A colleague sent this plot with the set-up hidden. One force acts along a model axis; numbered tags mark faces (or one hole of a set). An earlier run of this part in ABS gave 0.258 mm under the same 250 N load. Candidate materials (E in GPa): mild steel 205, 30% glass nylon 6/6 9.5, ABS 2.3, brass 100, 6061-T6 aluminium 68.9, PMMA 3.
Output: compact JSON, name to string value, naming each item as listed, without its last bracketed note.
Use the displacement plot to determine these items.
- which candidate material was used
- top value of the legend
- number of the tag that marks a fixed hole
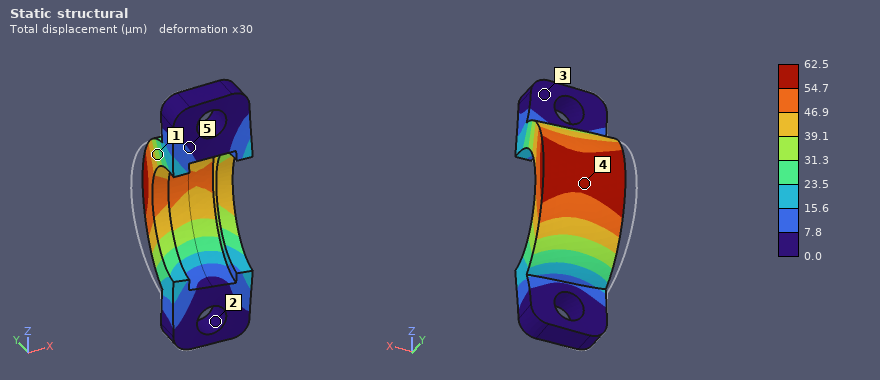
{"which candidate material was used": "30% glass nylon 6/6", "top value of the legend": "62.5 µm", "number of the tag that marks a fixed hole": "2"}
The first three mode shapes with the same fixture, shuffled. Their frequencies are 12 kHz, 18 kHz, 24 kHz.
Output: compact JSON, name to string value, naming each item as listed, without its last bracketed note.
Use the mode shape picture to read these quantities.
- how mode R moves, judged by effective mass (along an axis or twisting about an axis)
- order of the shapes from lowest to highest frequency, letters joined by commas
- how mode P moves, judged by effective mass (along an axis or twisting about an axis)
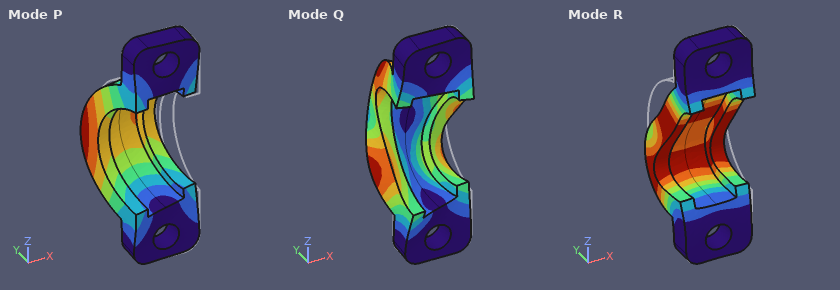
{"how mode R moves, judged by effective mass": "along Z", "order of the shapes from lowest to highest frequency, letters joined by commas": "P, R, Q", "how mode P moves, judged by effective mass": "along X"}
